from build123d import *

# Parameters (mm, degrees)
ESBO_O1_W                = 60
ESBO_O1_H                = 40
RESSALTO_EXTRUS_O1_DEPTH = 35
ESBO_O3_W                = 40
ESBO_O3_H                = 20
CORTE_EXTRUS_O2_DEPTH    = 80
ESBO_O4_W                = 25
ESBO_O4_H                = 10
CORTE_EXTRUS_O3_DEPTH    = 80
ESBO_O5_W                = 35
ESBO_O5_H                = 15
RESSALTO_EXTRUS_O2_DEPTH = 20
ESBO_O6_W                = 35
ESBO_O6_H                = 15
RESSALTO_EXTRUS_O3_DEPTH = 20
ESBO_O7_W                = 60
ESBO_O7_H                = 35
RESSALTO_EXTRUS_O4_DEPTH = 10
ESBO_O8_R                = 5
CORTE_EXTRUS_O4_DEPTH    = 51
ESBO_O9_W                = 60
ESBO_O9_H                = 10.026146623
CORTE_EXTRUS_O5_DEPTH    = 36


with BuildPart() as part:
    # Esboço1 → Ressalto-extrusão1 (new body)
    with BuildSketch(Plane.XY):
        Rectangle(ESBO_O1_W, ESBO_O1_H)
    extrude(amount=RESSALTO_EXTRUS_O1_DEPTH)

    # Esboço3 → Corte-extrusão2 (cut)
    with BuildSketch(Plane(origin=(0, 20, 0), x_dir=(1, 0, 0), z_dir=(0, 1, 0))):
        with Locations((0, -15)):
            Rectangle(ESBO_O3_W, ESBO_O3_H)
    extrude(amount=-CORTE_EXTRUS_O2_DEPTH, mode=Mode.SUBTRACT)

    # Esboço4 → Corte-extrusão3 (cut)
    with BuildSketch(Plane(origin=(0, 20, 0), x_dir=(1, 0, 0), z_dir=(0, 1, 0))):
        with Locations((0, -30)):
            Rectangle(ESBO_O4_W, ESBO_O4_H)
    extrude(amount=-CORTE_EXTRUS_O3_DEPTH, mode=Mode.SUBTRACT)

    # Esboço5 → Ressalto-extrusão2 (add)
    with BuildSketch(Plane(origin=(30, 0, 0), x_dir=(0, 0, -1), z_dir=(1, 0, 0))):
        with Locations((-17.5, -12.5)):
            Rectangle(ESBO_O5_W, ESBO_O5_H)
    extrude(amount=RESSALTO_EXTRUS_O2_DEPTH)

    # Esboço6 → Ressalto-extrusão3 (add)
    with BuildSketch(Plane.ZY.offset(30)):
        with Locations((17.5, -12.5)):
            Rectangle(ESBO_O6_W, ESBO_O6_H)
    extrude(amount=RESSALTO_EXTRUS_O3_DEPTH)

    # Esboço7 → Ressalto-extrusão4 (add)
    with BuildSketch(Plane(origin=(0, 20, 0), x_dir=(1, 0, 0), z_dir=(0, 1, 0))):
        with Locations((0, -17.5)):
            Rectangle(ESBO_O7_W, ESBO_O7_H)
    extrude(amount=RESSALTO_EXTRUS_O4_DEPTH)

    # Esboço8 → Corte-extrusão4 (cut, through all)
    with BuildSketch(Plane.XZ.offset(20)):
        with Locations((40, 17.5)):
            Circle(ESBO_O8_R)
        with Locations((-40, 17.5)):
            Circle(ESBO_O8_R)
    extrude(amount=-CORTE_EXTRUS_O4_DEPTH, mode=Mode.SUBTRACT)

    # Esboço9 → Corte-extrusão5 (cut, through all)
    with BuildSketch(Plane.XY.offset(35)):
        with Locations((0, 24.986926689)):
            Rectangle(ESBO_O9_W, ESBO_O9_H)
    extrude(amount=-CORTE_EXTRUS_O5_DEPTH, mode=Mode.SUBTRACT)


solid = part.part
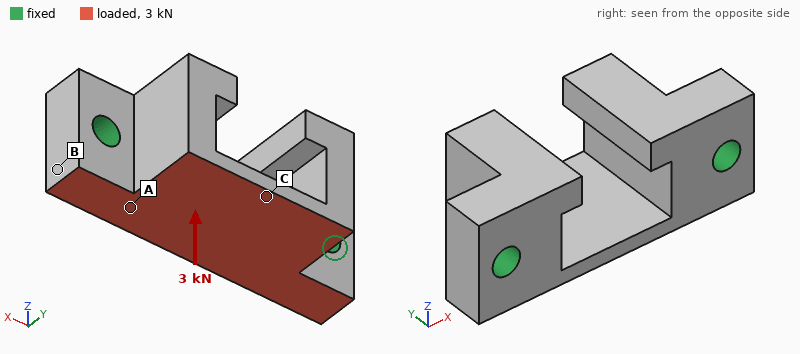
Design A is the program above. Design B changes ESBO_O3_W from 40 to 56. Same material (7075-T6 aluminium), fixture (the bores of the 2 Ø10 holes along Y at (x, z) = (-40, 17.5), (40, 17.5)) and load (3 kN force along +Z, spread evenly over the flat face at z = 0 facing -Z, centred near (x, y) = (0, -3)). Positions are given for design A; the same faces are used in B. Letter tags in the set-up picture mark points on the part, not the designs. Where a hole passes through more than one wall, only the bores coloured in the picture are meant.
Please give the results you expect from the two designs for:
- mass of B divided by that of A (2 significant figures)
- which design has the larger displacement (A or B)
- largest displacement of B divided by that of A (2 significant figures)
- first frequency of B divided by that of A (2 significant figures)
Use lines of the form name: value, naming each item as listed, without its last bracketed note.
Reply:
mass of B divided by that of A: 0.79
which design has the larger displacement: B
largest displacement of B divided by that of A: 4.0
first frequency of B divided by that of A: 0.69
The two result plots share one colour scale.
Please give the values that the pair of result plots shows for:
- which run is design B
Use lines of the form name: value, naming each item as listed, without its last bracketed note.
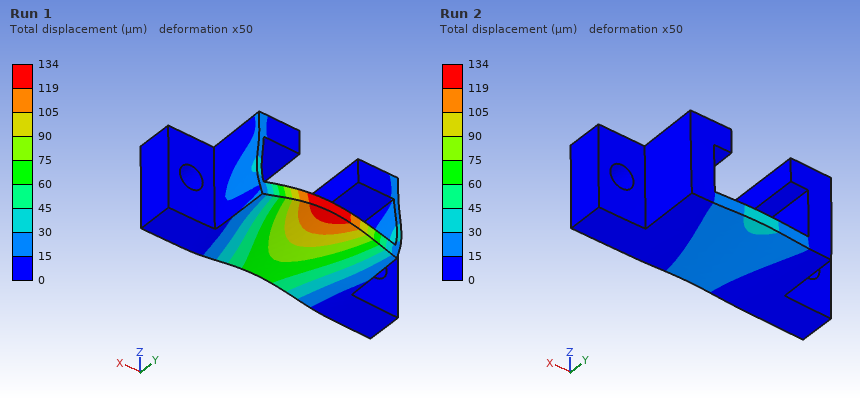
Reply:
which run is design B: Run 1
